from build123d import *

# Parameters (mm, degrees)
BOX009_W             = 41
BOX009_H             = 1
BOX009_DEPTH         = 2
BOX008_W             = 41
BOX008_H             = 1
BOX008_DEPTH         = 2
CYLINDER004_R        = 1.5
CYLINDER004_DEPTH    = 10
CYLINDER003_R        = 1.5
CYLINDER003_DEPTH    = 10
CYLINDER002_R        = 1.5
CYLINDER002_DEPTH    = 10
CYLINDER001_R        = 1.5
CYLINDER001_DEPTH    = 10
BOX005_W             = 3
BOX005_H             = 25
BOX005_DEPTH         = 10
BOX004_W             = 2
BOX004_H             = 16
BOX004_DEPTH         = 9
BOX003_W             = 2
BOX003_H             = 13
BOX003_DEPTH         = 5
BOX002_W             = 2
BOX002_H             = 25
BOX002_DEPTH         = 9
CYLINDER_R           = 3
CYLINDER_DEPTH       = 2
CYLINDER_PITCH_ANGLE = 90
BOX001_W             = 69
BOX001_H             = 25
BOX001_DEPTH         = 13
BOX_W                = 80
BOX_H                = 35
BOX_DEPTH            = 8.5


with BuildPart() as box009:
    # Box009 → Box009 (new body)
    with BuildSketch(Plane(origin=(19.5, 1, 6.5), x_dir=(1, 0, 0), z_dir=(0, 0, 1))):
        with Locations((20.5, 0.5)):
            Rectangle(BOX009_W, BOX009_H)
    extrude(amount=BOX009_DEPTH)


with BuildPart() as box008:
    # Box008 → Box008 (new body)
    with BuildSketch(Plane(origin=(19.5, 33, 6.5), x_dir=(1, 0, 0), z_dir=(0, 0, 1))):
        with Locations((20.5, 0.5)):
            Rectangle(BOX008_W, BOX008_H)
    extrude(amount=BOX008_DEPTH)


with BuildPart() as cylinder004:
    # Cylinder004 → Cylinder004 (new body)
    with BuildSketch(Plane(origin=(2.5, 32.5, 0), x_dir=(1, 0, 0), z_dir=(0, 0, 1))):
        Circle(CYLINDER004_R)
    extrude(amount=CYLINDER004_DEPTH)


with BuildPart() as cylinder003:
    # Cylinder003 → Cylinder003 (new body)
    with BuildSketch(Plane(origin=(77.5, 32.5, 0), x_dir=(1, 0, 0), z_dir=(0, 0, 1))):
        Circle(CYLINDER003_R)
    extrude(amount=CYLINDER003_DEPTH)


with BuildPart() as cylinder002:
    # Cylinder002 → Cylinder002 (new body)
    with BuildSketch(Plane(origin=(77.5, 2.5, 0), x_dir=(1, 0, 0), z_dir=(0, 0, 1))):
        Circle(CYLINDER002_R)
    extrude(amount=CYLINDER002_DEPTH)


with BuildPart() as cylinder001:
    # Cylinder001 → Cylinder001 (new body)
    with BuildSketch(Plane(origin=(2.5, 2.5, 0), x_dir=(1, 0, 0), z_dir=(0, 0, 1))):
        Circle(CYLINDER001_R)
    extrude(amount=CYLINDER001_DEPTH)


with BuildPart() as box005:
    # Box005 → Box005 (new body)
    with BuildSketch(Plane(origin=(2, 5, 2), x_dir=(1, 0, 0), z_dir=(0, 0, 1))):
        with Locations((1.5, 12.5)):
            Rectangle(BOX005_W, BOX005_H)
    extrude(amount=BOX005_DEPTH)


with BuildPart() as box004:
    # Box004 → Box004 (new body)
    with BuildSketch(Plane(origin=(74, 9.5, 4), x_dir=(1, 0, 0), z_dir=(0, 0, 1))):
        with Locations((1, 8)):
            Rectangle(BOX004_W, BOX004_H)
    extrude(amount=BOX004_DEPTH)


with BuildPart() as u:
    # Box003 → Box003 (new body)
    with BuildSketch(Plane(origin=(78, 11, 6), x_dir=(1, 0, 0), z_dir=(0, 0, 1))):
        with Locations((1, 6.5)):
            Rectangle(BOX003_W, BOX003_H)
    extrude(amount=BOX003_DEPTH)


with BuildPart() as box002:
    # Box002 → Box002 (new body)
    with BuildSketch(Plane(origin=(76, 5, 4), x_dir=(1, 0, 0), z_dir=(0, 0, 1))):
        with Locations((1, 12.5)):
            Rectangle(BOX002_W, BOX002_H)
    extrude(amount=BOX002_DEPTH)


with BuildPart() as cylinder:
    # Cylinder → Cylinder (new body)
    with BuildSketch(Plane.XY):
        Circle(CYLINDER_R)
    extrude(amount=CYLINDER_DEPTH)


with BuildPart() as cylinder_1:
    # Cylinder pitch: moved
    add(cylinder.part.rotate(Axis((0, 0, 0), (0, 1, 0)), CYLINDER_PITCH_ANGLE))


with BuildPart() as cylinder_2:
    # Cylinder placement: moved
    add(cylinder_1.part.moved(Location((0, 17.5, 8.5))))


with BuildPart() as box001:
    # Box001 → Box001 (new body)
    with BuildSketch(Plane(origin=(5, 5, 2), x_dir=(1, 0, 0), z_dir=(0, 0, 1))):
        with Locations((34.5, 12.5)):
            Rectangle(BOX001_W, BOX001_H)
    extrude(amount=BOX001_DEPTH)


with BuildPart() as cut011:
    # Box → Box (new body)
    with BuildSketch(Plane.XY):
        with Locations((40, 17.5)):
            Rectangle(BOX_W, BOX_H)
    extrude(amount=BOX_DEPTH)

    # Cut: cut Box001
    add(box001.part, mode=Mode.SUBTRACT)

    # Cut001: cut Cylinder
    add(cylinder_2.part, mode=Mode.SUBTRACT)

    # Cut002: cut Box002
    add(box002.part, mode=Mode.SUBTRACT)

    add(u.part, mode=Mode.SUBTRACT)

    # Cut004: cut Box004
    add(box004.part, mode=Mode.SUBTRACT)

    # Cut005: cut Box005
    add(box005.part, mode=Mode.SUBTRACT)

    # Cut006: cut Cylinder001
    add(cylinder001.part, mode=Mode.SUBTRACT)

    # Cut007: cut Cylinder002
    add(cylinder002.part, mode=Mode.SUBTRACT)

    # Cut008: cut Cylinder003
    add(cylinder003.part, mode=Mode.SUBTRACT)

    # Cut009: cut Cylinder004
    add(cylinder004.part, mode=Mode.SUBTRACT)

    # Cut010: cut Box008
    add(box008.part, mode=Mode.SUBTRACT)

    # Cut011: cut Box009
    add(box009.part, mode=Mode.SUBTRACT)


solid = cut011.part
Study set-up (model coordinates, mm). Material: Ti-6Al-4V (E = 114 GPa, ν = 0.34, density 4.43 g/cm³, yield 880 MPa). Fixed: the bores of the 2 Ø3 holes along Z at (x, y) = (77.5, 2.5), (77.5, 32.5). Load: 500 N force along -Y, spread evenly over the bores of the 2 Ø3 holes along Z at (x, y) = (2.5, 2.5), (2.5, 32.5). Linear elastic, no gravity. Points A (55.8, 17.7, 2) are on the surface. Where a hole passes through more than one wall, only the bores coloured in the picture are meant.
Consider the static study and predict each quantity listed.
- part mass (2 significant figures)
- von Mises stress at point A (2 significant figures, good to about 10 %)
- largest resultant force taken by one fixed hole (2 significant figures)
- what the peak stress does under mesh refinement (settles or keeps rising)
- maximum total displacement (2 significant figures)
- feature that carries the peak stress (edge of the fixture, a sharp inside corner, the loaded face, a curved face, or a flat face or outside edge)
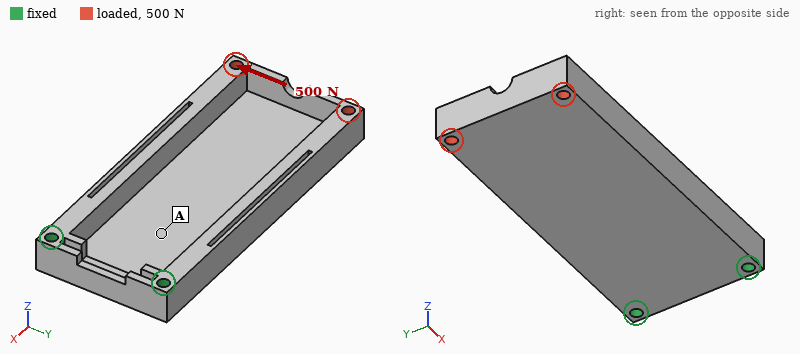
50 g
27 MPa
1.2 kN
keeps rising
0.16 mm
edge of the fixture
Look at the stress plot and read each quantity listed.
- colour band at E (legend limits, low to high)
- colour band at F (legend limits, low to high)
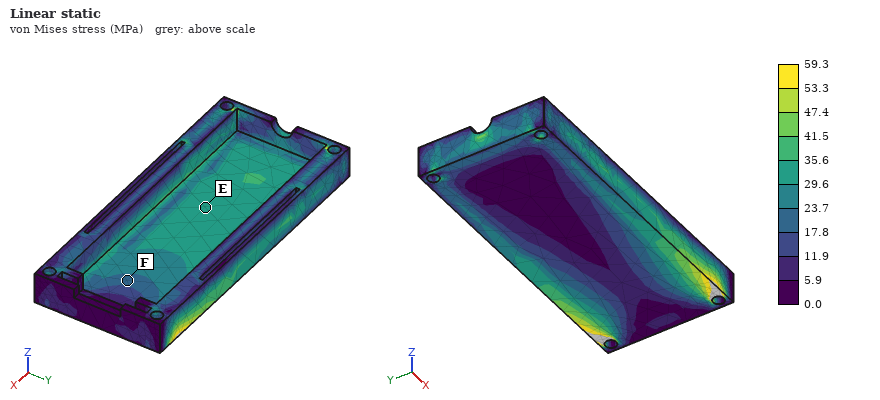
29.6 to 35.6 MPa
17.8 to 23.7 MPa
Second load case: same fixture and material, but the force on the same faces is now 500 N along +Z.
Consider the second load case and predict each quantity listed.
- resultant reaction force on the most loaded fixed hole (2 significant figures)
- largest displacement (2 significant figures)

670 N
0.87 mm
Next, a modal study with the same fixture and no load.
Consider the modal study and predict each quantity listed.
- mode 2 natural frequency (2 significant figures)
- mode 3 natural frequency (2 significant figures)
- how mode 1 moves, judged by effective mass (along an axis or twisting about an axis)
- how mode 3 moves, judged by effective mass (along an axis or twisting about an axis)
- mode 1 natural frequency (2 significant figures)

2000 Hz
4800 Hz
along Z
along Y
1100 Hz
